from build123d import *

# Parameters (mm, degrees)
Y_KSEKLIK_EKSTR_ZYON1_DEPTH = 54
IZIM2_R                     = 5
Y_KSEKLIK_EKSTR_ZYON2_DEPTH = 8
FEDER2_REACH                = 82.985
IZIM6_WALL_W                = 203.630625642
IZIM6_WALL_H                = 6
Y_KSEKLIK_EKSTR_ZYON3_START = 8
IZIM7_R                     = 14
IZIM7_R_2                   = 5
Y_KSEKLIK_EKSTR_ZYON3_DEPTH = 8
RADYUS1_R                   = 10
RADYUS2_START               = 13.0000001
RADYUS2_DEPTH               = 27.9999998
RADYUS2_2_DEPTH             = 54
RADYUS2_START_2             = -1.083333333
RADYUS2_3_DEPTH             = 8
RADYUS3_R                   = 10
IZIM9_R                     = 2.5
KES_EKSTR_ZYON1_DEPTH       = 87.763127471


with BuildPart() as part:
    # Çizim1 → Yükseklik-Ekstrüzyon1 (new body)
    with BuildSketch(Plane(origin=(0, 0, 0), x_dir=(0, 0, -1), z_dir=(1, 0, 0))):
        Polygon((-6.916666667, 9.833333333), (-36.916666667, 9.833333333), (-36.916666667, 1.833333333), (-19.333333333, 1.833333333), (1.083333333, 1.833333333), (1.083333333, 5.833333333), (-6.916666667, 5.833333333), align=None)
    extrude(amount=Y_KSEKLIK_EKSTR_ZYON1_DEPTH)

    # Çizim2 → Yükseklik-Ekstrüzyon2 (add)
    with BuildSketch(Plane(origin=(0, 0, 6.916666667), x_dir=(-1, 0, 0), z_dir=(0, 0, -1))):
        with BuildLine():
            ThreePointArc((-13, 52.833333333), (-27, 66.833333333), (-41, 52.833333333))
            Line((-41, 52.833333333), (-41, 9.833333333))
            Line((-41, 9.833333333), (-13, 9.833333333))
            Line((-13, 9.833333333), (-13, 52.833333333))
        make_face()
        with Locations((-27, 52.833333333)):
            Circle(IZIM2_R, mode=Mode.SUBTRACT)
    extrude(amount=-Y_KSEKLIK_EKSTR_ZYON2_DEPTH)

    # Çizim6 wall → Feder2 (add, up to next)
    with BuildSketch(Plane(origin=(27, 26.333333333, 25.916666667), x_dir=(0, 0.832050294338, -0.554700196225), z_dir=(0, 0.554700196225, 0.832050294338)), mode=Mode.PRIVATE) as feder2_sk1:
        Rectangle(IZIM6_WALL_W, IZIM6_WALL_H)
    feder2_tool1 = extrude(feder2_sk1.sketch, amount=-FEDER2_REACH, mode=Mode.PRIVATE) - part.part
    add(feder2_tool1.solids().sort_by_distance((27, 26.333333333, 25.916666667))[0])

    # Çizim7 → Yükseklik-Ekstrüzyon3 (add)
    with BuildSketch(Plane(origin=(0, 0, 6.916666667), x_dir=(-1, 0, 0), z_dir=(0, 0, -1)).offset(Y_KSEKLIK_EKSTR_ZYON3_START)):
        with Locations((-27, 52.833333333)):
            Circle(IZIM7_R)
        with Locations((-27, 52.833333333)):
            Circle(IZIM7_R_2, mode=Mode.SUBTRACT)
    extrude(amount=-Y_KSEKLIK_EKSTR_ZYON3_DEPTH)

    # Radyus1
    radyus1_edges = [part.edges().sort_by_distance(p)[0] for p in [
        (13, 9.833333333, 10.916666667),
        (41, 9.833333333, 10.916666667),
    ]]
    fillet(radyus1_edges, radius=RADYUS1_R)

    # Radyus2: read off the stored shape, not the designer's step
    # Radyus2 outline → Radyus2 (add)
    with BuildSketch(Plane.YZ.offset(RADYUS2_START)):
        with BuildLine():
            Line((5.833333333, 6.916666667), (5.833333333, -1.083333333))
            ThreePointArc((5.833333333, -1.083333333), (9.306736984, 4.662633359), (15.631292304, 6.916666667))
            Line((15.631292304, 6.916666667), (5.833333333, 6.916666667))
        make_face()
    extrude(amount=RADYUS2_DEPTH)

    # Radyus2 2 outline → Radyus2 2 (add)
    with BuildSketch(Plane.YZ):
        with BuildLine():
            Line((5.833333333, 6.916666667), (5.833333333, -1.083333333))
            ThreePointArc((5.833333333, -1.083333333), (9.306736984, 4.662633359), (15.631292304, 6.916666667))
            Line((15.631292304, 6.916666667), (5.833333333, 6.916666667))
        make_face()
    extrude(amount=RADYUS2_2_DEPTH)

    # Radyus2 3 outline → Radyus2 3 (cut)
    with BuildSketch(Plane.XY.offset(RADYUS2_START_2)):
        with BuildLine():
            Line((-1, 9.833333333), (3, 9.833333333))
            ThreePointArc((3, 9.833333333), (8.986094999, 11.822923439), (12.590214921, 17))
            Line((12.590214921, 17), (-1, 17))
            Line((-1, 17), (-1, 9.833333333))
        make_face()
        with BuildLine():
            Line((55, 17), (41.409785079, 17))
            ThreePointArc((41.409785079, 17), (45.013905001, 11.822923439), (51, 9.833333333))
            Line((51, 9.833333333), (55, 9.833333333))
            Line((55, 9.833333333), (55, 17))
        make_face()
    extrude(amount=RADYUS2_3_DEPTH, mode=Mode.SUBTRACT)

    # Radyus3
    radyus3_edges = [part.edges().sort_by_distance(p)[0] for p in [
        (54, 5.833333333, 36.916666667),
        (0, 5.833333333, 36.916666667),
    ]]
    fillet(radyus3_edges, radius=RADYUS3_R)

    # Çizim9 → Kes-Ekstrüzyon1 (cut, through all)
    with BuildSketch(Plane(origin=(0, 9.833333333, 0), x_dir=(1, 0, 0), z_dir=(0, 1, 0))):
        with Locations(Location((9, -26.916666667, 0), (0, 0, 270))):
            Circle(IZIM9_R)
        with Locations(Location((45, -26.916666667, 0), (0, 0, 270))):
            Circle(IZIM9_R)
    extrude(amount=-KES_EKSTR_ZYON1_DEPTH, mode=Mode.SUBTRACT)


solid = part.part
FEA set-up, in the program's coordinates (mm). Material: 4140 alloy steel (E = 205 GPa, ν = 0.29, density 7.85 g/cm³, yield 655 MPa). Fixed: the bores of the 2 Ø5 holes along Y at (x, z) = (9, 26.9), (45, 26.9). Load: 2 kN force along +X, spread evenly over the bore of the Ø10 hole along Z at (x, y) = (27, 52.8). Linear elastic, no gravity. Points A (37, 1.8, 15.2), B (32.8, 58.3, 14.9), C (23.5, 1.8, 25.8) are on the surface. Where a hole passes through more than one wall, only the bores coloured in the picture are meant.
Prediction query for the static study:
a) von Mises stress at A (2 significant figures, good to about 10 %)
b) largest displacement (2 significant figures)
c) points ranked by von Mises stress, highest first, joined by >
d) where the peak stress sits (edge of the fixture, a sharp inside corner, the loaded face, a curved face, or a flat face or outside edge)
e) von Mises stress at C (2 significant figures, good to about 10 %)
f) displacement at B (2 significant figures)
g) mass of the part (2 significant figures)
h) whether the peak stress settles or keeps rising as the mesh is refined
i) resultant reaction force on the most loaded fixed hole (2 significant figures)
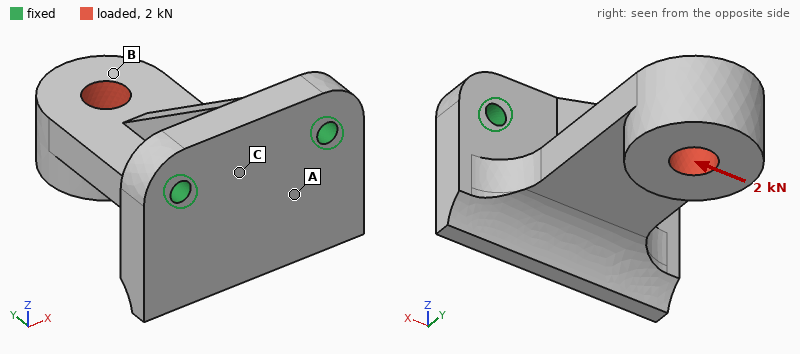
42 MPa
70 µm
A > C > B
edge of the fixture
26 MPa
54 µm
260 g
keeps rising
3.0 kN
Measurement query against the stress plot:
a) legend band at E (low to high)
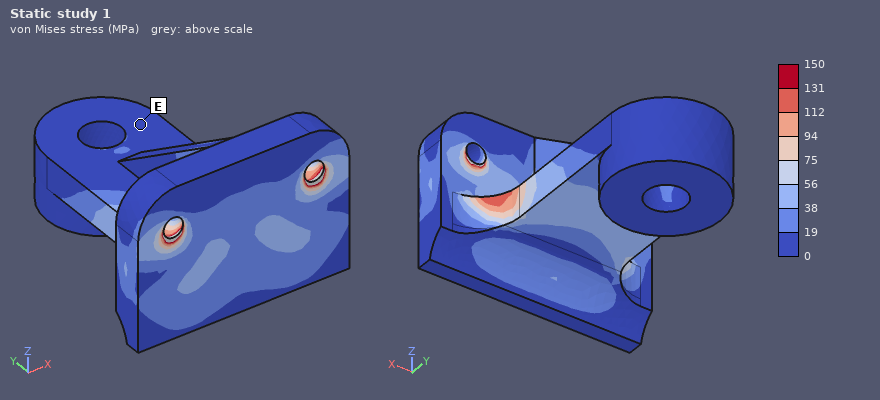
0 to 19 MPa
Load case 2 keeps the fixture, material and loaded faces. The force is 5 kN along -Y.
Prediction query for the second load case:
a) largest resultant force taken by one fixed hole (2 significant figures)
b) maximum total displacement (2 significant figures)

2.5 kN
0.16 mm
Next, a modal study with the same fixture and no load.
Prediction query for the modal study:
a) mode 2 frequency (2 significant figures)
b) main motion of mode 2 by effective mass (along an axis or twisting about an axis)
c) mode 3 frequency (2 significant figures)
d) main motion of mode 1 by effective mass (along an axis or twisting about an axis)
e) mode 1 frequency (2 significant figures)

3400 Hz
along X
7100 Hz
along Z
2000 Hz
